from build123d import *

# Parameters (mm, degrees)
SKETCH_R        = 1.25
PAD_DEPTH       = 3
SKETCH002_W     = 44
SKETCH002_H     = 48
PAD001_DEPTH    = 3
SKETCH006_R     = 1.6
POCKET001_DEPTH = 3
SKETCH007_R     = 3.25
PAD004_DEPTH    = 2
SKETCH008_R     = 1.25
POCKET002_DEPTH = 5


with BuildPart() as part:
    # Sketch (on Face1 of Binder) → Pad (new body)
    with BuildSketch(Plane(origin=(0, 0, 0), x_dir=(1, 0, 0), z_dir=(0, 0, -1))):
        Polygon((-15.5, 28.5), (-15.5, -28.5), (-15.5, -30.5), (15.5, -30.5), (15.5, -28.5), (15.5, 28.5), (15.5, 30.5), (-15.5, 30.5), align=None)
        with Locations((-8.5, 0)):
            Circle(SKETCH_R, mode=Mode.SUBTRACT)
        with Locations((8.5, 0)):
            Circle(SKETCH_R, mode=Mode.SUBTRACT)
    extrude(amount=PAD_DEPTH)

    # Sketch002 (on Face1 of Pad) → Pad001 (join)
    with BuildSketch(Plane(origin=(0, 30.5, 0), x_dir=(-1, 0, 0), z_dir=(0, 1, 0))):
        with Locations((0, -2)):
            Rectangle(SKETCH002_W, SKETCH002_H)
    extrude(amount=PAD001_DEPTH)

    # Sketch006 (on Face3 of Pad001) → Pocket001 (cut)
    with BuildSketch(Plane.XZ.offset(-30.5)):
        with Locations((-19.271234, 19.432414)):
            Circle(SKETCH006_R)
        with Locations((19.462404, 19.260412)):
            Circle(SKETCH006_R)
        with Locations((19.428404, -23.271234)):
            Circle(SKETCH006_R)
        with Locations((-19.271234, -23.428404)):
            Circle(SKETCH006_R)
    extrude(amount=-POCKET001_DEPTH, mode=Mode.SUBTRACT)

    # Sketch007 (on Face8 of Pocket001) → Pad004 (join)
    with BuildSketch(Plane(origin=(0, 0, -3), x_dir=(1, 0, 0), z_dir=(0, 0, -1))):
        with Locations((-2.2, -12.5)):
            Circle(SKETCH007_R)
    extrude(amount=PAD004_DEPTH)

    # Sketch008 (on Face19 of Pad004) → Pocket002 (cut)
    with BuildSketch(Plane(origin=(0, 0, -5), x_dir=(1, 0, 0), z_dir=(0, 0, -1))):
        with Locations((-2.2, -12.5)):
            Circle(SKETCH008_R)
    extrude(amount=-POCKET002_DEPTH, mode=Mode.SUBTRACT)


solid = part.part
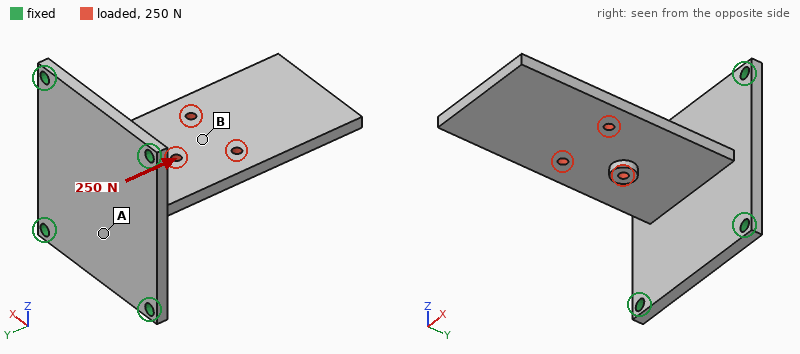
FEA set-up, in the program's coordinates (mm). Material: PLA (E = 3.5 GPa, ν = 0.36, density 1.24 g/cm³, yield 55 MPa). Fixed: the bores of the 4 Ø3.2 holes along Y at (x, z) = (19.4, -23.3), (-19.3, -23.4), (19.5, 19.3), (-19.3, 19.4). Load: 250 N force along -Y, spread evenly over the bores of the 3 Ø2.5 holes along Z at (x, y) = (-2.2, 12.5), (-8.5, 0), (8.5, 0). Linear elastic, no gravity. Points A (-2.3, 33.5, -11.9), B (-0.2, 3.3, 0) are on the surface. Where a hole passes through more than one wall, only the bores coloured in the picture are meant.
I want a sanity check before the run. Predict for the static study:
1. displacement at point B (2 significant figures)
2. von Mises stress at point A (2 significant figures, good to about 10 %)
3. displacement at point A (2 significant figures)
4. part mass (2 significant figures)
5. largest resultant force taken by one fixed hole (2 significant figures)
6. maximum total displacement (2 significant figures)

0.47 mm
7.1 MPa
0.33 mm
15 g
67 N
0.73 mm
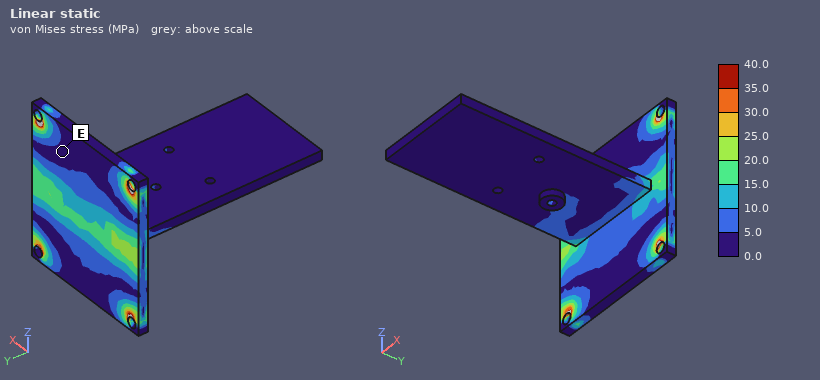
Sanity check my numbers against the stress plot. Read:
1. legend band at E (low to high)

0.0 to 5.0 MPa
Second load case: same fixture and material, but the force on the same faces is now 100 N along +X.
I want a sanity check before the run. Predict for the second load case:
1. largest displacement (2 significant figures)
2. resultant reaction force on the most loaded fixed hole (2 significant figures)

1.00 mm
49 N
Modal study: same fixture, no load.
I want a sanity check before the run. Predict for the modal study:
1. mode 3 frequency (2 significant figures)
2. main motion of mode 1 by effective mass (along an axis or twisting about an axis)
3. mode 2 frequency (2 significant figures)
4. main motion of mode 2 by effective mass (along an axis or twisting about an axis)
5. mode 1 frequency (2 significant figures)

880 Hz
along Z
640 Hz
along X
210 Hz
